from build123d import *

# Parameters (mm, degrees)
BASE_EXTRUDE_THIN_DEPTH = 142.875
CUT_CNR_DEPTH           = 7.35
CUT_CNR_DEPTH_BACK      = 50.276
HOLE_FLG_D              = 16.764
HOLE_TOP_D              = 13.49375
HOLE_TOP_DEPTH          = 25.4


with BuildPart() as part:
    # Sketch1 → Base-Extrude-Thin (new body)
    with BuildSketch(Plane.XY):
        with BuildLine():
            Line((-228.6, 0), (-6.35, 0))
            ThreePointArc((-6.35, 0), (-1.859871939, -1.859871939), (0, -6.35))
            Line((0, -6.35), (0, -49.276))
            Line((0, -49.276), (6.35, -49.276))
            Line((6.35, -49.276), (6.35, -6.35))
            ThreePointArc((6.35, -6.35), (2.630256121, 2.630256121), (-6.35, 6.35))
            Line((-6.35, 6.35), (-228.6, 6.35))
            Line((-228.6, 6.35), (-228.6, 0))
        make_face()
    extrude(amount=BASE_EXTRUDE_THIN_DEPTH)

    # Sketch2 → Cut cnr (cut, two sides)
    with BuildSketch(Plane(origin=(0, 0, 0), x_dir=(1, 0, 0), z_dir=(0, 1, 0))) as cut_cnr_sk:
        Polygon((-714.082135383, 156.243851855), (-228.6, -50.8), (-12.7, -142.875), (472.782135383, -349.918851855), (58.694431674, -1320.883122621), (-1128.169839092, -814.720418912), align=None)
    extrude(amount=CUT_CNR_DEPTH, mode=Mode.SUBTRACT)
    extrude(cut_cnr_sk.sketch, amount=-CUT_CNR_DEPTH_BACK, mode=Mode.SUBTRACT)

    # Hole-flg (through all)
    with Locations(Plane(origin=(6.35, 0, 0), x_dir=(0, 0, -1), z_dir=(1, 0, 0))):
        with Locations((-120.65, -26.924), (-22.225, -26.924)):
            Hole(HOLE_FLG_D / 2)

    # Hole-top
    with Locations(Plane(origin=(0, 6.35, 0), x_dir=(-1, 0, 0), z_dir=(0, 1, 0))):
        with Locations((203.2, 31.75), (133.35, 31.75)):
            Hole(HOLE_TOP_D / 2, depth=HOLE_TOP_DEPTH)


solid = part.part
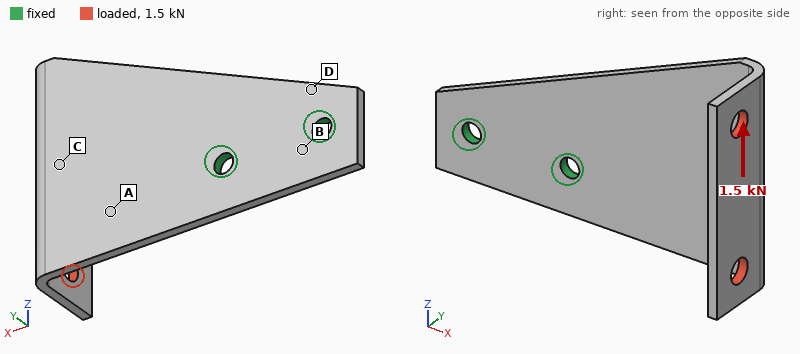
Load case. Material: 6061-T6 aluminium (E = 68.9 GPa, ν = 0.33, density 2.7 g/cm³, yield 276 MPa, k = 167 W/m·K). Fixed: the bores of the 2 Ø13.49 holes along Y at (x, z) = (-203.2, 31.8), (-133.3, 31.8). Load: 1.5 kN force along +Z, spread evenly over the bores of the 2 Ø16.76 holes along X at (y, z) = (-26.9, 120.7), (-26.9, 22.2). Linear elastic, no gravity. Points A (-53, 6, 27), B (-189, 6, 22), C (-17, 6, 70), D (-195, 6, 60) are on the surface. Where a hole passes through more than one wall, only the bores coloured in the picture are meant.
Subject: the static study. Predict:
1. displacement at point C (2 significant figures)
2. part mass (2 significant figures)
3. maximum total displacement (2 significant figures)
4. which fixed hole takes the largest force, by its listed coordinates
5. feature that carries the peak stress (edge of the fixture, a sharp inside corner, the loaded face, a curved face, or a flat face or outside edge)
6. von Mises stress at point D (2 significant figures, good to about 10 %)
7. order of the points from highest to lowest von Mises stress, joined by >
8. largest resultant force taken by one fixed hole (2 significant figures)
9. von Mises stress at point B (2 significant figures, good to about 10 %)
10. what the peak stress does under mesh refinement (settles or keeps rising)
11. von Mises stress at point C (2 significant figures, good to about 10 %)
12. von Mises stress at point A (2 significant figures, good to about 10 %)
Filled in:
0.66 mm
500 g
2.9 mm
(-133.3, 31.8)
edge of the fixture
20 MPa
A > C > D > B
3.9 kN
9.9 MPa
keeps rising
28 MPa
47 MPa
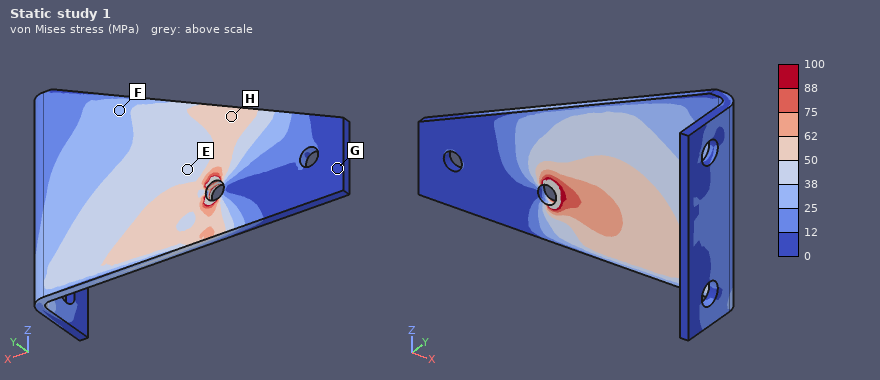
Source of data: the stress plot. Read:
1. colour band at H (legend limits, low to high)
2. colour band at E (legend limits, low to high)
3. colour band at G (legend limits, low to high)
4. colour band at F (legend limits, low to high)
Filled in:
50 to 62 MPa
38 to 50 MPa
0 to 12 MPa
25 to 38 MPa
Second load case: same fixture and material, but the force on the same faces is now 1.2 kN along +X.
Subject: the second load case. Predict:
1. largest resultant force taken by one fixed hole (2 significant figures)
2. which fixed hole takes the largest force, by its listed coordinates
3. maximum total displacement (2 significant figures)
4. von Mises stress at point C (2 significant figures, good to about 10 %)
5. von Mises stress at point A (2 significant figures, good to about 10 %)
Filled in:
960 N
(-133.3, 31.8)
3.0 mm
34 MPa
41 MPa
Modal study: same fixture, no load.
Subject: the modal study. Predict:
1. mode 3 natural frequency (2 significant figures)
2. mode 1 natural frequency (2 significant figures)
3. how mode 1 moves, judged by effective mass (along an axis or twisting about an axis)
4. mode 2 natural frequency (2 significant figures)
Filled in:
770 Hz
140 Hz
along Y
320 Hz
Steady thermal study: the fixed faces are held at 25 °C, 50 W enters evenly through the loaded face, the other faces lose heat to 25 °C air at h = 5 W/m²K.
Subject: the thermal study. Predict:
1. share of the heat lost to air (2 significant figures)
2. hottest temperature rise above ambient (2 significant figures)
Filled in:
20 %
69 K
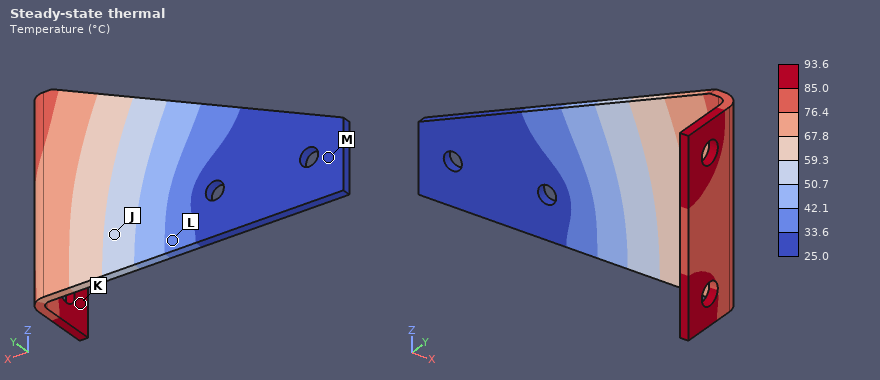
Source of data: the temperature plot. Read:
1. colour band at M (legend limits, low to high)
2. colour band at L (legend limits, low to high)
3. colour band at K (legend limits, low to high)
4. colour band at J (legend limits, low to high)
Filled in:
25.0 to 33.6 °C
33.6 to 42.1 °C
85.0 to 93.6 °C
50.7 to 59.3 °C
